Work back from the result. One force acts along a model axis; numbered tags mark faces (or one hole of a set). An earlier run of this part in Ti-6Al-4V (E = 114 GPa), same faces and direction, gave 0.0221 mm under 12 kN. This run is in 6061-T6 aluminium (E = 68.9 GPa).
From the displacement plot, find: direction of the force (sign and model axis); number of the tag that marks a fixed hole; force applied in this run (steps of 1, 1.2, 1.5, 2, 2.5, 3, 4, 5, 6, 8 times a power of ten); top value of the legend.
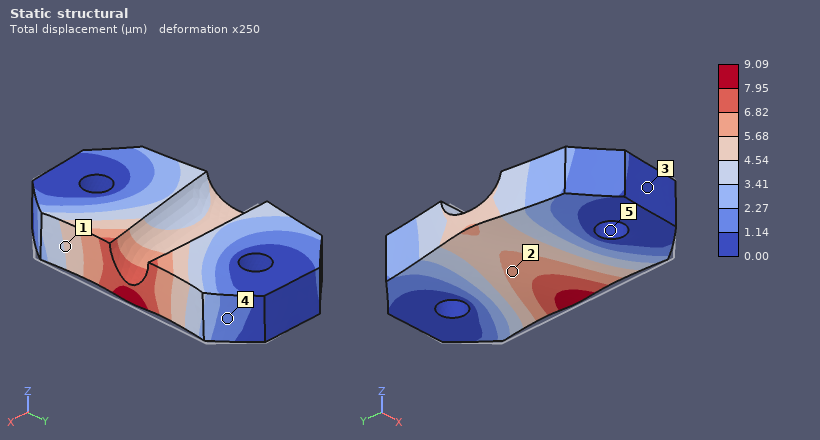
-X
5
3 kN
9.09 µm
